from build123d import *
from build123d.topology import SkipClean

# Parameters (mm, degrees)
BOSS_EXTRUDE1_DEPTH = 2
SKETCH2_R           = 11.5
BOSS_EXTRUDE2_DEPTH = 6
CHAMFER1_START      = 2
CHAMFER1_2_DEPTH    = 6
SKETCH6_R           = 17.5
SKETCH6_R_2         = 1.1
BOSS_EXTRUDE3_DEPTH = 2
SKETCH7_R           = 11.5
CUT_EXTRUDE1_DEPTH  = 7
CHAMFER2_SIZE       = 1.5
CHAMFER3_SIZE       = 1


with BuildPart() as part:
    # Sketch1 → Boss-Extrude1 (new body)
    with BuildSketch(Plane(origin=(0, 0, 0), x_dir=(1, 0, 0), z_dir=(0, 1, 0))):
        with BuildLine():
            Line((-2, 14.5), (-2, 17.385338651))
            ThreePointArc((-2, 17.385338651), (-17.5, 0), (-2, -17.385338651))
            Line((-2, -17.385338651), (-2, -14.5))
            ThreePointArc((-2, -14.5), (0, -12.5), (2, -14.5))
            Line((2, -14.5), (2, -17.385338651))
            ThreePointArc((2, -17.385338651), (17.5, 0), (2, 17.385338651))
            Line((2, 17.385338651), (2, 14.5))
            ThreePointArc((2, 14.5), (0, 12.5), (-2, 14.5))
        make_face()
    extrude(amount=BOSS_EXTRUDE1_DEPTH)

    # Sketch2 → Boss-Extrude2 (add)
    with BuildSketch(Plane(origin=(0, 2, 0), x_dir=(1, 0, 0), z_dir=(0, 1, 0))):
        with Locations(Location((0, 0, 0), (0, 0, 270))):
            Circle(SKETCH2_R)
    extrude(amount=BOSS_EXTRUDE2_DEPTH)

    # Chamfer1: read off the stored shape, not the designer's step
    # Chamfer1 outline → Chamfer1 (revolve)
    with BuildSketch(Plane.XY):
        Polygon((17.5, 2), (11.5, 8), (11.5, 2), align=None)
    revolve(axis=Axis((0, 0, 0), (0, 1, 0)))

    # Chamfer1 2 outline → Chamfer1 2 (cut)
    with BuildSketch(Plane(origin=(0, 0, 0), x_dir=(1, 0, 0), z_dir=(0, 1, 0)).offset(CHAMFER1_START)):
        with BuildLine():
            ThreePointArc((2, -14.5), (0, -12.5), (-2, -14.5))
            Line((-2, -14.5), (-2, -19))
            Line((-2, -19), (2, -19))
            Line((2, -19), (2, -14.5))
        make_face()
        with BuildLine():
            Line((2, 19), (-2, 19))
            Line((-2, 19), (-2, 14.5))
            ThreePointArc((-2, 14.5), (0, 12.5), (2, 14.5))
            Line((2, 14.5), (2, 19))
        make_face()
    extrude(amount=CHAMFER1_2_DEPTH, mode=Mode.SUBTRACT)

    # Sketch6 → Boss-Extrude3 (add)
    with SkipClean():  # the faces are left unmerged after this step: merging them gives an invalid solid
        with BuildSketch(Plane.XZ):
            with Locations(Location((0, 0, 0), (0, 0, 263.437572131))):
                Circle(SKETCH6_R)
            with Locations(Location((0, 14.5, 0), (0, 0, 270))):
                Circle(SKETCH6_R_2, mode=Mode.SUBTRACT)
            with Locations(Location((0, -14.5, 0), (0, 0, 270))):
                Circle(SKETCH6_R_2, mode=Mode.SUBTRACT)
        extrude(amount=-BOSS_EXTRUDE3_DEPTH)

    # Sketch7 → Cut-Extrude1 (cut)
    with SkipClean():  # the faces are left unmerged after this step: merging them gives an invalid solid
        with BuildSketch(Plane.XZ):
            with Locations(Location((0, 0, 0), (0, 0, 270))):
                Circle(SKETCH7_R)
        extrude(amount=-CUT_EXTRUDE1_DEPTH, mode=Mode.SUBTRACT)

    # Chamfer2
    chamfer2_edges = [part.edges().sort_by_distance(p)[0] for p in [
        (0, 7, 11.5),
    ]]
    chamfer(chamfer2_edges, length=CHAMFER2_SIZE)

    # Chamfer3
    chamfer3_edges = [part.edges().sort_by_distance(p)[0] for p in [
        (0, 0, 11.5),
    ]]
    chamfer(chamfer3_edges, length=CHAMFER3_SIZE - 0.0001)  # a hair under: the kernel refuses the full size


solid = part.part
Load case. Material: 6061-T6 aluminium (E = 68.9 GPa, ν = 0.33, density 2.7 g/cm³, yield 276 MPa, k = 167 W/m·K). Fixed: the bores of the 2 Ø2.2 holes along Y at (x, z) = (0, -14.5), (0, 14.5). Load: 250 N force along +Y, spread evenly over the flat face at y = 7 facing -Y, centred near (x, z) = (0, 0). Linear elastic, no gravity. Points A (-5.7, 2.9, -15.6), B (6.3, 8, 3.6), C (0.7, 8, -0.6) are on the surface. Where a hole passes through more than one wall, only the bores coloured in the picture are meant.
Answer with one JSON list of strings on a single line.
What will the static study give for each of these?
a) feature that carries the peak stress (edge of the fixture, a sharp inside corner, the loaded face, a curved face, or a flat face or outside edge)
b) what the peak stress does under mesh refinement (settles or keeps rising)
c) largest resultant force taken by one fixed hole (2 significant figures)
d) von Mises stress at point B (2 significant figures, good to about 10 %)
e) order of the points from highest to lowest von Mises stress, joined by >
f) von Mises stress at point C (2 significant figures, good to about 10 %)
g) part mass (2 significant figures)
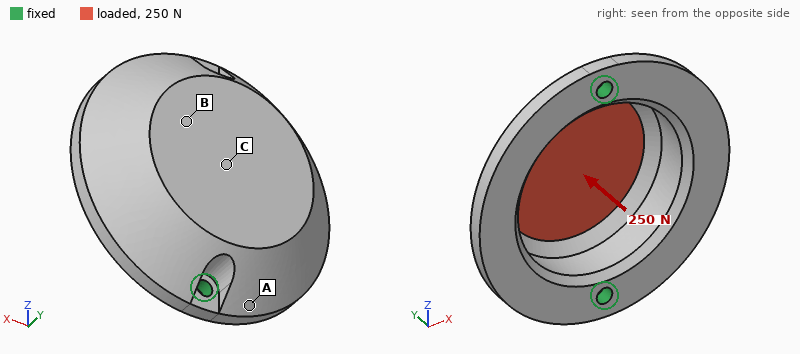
["edge of the fixture", "keeps rising", "160 N", "24 MPa", "C > B > A", "51 MPa", "8.0 g"]
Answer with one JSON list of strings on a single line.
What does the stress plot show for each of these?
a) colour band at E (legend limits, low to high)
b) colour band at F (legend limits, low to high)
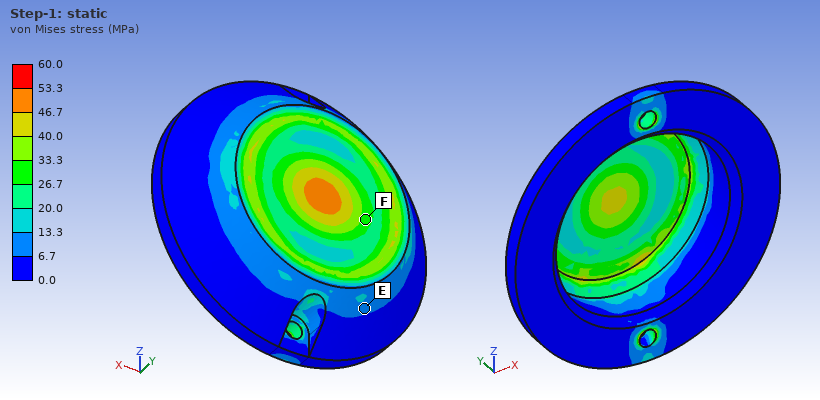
["6.7 to 13.3 MPa", "26.7 to 33.3 MPa"]
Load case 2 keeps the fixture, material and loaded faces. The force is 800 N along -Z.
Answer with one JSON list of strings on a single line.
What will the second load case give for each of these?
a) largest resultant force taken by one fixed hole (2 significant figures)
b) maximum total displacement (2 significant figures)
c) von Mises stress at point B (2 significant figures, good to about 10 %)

["420 N", "14 µm", "11 MPa"]
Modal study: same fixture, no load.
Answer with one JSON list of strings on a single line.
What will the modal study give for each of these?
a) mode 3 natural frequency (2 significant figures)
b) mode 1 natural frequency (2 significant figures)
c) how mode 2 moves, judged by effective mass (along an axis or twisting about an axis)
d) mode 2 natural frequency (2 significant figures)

["15 kHz", "4900 Hz", "along Y", "14 kHz"]
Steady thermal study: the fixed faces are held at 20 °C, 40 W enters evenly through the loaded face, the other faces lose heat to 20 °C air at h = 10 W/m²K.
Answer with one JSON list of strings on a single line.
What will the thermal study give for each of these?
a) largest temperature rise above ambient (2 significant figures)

["52 K"]
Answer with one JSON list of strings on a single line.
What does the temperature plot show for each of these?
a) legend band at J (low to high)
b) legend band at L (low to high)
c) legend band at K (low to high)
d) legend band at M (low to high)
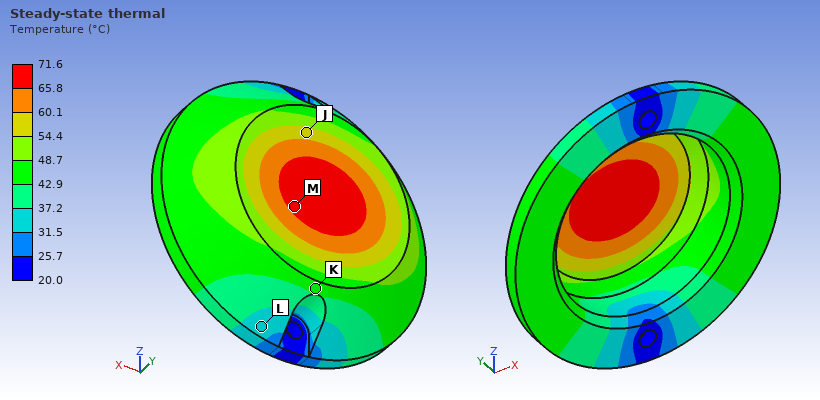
["54.4 to 60.1 °C", "31.5 to 37.2 °C", "42.9 to 48.7 °C", "65.8 to 71.6 °C"]
